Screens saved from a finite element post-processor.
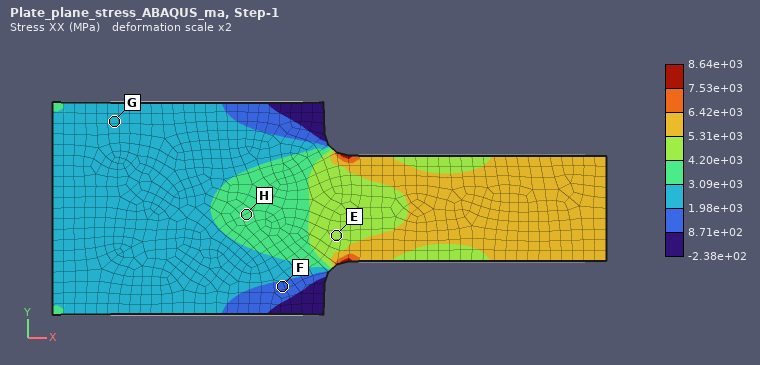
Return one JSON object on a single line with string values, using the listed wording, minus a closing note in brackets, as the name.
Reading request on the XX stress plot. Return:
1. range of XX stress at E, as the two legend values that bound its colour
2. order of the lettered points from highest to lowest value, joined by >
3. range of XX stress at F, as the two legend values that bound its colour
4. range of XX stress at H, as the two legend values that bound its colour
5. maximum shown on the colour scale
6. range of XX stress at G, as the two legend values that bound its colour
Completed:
{"range of XX stress at E, as the two legend values that bound its colour": "4.20e+03 to 5.31e+03 MPa", "order of the lettered points from highest to lowest value, joined by >": "E > H > G > F", "range of XX stress at F, as the two legend values that bound its colour": "8.71e+02 to 1.98e+03 MPa", "range of XX stress at H, as the two legend values that bound its colour": "3.09e+03 to 4.20e+03 MPa", "maximum shown on the colour scale": "8.64e+03 MPa", "range of XX stress at G, as the two legend values that bound its colour": "1.98e+03 to 3.09e+03 MPa"}
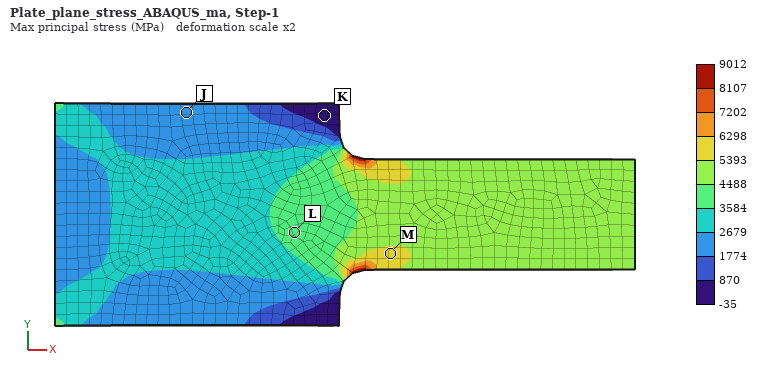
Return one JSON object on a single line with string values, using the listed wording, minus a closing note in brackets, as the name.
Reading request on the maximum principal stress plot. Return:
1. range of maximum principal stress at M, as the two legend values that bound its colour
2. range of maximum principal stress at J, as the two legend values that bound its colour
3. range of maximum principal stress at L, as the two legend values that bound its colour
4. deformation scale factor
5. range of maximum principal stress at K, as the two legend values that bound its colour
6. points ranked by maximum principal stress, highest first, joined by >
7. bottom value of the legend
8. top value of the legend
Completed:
{"range of maximum principal stress at M, as the two legend values that bound its colour": "5393 to 6298 MPa", "range of maximum principal stress at J, as the two legend values that bound its colour": "1774 to 2679 MPa", "range of maximum principal stress at L, as the two legend values that bound its colour": "3584 to 4488 MPa", "deformation scale factor": "2", "range of maximum principal stress at K, as the two legend values that bound its colour": "-35 to 870 MPa", "points ranked by maximum principal stress, highest first, joined by >": "M > L > J > K", "bottom value of the legend": "-35 MPa", "top value of the legend": "9012 MPa"}
